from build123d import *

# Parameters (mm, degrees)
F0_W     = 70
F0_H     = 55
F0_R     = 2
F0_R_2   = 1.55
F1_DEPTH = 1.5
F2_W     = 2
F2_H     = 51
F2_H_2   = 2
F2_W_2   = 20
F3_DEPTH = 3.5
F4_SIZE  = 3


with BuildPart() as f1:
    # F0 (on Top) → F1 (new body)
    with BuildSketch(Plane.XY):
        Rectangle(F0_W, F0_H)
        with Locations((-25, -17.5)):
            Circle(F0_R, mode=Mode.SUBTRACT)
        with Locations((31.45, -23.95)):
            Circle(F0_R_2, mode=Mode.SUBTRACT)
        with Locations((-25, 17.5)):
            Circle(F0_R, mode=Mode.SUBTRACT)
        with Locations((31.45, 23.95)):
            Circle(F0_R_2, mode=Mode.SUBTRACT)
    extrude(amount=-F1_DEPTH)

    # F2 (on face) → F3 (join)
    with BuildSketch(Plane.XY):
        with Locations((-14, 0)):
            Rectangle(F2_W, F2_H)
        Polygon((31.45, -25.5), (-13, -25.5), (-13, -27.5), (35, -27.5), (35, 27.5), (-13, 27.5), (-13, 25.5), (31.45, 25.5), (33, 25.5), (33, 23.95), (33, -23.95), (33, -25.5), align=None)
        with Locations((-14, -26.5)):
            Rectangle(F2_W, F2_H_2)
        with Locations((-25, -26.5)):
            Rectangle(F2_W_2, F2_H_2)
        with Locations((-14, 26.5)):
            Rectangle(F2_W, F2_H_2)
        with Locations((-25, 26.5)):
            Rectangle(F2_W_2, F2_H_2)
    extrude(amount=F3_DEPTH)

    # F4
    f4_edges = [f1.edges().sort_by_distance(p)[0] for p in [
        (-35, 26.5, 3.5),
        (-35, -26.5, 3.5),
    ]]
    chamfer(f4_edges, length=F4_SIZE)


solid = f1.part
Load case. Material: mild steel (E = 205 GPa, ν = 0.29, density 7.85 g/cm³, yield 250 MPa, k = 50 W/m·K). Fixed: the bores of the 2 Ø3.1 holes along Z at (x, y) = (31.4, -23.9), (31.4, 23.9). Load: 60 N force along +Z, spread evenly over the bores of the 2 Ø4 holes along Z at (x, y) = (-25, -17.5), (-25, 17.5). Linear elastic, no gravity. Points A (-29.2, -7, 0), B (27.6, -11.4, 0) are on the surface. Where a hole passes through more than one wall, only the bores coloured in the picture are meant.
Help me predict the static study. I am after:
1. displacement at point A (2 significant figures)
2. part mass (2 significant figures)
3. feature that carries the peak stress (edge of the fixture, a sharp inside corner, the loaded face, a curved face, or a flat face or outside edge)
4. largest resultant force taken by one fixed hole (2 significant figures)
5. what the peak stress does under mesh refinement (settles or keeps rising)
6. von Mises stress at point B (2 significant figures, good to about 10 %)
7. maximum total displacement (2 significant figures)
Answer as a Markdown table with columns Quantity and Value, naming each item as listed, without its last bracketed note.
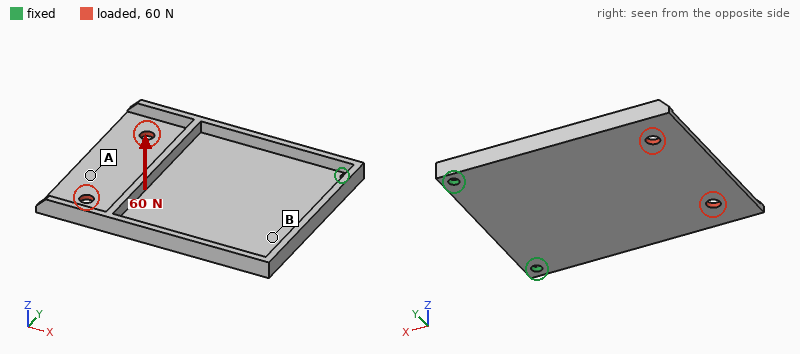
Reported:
| Quantity | Value |
|---|---|
| displacement at point A | 0.30 mm |
| part mass | 58 g |
| feature that carries the peak stress | edge of the fixture |
| largest resultant force taken by one fixed hole | 100 N |
| what the peak stress does under mesh refinement | keeps rising |
| von Mises stress at point B | 23 MPa |
| maximum total displacement | 0.34 mm |
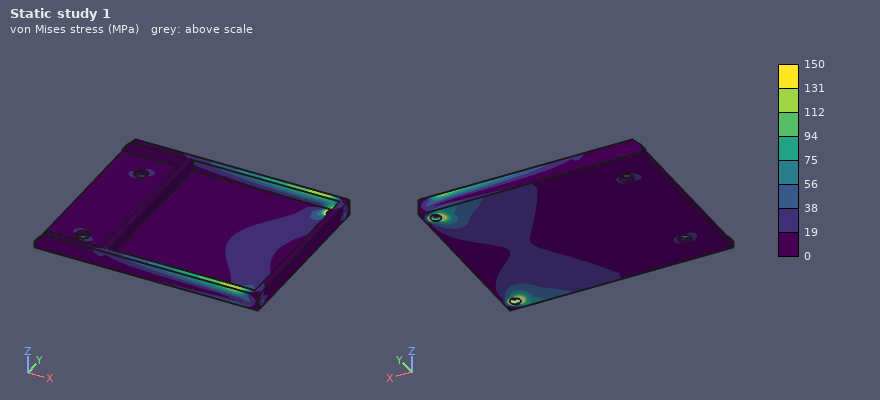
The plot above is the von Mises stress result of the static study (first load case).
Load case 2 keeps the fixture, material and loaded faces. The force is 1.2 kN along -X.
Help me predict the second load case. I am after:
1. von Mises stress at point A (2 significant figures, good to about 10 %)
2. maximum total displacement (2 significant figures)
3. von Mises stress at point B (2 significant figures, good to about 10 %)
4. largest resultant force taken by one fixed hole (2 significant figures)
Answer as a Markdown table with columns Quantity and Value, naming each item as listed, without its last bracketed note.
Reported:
| Quantity | Value |
|---|---|
| von Mises stress at point A | 7.2 MPa |
| maximum total displacement | 68 µm |
| von Mises stress at point B | 8.5 MPa |
| largest resultant force taken by one fixed hole | 620 N |
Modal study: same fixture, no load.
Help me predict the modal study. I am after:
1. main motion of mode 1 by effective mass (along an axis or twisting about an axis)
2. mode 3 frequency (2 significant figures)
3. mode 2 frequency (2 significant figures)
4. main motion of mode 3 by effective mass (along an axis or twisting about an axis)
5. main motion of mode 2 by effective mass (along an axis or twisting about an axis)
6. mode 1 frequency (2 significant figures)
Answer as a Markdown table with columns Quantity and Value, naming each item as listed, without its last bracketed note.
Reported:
| Quantity | Value |
|---|---|
| main motion of mode 1 by effective mass | along Z |
| mode 3 frequency | 2700 Hz |
| mode 2 frequency | 1000 Hz |
| main motion of mode 3 by effective mass | along Z |
| main motion of mode 2 by effective mass | twisting about X |
| mode 1 frequency | 510 Hz |
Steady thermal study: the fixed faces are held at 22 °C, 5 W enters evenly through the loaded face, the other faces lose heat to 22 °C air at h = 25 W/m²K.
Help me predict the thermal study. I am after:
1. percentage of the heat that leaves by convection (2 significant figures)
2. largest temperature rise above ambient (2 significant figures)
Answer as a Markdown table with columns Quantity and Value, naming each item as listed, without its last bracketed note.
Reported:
| Quantity | Value |
|---|---|
| percentage of the heat that leaves by convection | 71 % |
| largest temperature rise above ambient | 36 K |
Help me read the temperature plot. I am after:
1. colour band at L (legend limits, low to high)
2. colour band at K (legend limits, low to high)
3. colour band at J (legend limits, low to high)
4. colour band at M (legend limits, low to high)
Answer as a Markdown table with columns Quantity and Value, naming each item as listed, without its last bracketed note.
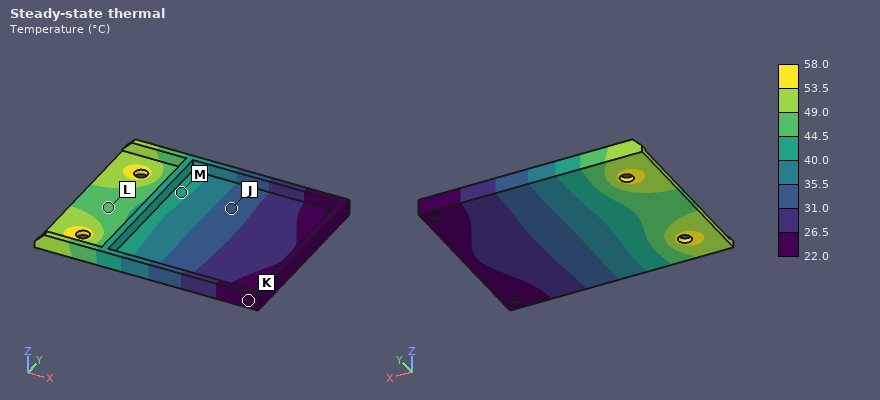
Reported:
| Quantity | Value |
|---|---|
| colour band at L | 44.5 to 49.0 °C |
| colour band at K | 22.0 to 26.5 °C |
| colour band at J | 31.0 to 35.5 °C |
| colour band at M | 40.0 to 44.5 °C |
